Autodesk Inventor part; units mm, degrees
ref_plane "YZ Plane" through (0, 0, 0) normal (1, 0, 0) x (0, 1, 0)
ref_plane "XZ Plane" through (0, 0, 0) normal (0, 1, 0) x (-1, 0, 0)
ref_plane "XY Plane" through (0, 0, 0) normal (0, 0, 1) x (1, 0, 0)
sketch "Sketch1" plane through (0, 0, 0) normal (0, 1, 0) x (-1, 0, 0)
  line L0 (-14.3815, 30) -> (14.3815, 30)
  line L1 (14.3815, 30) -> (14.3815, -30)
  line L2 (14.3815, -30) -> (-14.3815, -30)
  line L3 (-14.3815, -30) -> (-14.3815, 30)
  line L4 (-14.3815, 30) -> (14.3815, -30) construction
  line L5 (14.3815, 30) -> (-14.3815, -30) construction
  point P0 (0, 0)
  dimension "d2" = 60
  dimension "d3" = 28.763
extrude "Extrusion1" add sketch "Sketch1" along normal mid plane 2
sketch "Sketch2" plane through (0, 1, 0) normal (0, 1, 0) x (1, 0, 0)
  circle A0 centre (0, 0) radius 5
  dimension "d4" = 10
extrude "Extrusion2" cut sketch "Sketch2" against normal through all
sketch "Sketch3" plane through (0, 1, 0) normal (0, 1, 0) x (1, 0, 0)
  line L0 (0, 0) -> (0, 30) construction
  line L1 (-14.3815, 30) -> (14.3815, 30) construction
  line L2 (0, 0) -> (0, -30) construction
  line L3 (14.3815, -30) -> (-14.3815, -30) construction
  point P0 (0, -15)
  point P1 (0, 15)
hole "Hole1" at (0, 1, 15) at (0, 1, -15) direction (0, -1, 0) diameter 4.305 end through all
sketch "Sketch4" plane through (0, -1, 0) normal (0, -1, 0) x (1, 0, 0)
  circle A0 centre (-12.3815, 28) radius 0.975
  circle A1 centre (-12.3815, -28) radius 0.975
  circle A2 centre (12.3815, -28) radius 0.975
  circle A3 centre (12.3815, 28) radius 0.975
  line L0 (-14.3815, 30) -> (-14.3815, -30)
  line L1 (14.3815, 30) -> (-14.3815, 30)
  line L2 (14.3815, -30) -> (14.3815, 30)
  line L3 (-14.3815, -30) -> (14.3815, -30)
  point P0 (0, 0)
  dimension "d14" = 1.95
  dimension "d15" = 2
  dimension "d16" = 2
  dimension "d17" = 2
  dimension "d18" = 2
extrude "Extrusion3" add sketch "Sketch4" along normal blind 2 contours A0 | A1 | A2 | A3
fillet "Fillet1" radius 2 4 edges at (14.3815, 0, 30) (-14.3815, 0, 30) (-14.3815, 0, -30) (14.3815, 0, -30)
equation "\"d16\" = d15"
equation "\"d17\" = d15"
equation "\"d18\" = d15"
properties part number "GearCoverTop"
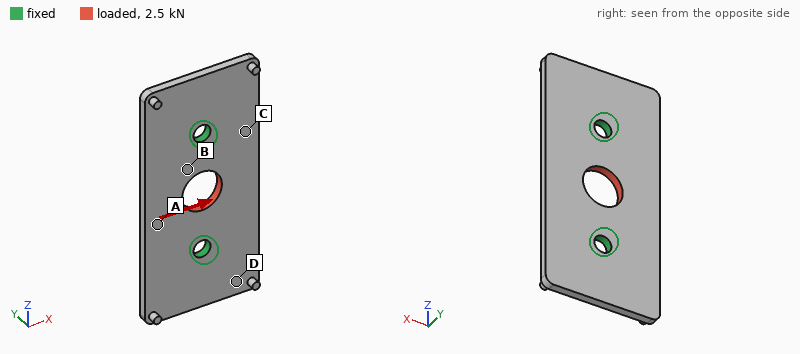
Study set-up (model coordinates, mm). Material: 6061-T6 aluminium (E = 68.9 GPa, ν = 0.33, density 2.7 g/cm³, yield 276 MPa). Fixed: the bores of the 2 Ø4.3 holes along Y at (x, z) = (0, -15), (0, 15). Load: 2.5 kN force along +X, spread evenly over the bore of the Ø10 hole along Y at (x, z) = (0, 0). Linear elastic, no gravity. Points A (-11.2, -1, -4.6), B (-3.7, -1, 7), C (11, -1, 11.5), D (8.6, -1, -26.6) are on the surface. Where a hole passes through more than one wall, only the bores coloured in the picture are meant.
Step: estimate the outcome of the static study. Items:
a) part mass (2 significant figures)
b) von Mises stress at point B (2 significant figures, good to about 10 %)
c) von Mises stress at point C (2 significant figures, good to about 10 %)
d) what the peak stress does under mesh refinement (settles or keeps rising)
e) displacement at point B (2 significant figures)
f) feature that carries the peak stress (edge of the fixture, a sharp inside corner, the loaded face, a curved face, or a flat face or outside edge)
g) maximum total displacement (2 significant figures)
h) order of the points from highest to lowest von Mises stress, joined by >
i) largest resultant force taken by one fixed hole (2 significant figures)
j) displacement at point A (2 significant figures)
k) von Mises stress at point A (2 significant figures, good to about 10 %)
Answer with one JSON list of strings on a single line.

["8.8 g", "50 MPa", "23 MPa", "keeps rising", "11 µm", "edge of the fixture", "18 µm", "B > A > C > D", "1.3 kN", "13 µm", "39 MPa"]
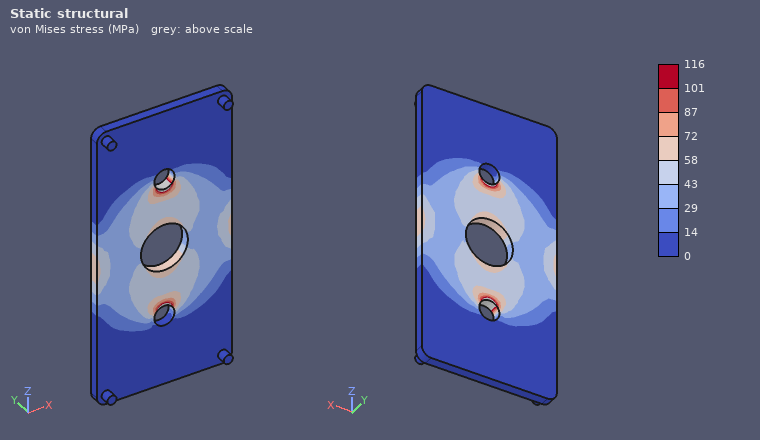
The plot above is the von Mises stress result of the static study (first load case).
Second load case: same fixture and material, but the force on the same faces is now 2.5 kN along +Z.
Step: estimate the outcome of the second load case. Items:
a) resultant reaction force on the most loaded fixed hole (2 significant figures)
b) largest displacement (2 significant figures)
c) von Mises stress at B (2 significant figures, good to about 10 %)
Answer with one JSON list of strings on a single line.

["1.3 kN", "9.0 µm", "45 MPa"]
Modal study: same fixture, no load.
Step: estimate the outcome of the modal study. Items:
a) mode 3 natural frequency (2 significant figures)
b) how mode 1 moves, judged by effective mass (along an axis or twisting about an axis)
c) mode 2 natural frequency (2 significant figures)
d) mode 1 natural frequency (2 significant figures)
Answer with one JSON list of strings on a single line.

["6600 Hz", "twisting about Z", "6500 Hz", "6200 Hz"]
